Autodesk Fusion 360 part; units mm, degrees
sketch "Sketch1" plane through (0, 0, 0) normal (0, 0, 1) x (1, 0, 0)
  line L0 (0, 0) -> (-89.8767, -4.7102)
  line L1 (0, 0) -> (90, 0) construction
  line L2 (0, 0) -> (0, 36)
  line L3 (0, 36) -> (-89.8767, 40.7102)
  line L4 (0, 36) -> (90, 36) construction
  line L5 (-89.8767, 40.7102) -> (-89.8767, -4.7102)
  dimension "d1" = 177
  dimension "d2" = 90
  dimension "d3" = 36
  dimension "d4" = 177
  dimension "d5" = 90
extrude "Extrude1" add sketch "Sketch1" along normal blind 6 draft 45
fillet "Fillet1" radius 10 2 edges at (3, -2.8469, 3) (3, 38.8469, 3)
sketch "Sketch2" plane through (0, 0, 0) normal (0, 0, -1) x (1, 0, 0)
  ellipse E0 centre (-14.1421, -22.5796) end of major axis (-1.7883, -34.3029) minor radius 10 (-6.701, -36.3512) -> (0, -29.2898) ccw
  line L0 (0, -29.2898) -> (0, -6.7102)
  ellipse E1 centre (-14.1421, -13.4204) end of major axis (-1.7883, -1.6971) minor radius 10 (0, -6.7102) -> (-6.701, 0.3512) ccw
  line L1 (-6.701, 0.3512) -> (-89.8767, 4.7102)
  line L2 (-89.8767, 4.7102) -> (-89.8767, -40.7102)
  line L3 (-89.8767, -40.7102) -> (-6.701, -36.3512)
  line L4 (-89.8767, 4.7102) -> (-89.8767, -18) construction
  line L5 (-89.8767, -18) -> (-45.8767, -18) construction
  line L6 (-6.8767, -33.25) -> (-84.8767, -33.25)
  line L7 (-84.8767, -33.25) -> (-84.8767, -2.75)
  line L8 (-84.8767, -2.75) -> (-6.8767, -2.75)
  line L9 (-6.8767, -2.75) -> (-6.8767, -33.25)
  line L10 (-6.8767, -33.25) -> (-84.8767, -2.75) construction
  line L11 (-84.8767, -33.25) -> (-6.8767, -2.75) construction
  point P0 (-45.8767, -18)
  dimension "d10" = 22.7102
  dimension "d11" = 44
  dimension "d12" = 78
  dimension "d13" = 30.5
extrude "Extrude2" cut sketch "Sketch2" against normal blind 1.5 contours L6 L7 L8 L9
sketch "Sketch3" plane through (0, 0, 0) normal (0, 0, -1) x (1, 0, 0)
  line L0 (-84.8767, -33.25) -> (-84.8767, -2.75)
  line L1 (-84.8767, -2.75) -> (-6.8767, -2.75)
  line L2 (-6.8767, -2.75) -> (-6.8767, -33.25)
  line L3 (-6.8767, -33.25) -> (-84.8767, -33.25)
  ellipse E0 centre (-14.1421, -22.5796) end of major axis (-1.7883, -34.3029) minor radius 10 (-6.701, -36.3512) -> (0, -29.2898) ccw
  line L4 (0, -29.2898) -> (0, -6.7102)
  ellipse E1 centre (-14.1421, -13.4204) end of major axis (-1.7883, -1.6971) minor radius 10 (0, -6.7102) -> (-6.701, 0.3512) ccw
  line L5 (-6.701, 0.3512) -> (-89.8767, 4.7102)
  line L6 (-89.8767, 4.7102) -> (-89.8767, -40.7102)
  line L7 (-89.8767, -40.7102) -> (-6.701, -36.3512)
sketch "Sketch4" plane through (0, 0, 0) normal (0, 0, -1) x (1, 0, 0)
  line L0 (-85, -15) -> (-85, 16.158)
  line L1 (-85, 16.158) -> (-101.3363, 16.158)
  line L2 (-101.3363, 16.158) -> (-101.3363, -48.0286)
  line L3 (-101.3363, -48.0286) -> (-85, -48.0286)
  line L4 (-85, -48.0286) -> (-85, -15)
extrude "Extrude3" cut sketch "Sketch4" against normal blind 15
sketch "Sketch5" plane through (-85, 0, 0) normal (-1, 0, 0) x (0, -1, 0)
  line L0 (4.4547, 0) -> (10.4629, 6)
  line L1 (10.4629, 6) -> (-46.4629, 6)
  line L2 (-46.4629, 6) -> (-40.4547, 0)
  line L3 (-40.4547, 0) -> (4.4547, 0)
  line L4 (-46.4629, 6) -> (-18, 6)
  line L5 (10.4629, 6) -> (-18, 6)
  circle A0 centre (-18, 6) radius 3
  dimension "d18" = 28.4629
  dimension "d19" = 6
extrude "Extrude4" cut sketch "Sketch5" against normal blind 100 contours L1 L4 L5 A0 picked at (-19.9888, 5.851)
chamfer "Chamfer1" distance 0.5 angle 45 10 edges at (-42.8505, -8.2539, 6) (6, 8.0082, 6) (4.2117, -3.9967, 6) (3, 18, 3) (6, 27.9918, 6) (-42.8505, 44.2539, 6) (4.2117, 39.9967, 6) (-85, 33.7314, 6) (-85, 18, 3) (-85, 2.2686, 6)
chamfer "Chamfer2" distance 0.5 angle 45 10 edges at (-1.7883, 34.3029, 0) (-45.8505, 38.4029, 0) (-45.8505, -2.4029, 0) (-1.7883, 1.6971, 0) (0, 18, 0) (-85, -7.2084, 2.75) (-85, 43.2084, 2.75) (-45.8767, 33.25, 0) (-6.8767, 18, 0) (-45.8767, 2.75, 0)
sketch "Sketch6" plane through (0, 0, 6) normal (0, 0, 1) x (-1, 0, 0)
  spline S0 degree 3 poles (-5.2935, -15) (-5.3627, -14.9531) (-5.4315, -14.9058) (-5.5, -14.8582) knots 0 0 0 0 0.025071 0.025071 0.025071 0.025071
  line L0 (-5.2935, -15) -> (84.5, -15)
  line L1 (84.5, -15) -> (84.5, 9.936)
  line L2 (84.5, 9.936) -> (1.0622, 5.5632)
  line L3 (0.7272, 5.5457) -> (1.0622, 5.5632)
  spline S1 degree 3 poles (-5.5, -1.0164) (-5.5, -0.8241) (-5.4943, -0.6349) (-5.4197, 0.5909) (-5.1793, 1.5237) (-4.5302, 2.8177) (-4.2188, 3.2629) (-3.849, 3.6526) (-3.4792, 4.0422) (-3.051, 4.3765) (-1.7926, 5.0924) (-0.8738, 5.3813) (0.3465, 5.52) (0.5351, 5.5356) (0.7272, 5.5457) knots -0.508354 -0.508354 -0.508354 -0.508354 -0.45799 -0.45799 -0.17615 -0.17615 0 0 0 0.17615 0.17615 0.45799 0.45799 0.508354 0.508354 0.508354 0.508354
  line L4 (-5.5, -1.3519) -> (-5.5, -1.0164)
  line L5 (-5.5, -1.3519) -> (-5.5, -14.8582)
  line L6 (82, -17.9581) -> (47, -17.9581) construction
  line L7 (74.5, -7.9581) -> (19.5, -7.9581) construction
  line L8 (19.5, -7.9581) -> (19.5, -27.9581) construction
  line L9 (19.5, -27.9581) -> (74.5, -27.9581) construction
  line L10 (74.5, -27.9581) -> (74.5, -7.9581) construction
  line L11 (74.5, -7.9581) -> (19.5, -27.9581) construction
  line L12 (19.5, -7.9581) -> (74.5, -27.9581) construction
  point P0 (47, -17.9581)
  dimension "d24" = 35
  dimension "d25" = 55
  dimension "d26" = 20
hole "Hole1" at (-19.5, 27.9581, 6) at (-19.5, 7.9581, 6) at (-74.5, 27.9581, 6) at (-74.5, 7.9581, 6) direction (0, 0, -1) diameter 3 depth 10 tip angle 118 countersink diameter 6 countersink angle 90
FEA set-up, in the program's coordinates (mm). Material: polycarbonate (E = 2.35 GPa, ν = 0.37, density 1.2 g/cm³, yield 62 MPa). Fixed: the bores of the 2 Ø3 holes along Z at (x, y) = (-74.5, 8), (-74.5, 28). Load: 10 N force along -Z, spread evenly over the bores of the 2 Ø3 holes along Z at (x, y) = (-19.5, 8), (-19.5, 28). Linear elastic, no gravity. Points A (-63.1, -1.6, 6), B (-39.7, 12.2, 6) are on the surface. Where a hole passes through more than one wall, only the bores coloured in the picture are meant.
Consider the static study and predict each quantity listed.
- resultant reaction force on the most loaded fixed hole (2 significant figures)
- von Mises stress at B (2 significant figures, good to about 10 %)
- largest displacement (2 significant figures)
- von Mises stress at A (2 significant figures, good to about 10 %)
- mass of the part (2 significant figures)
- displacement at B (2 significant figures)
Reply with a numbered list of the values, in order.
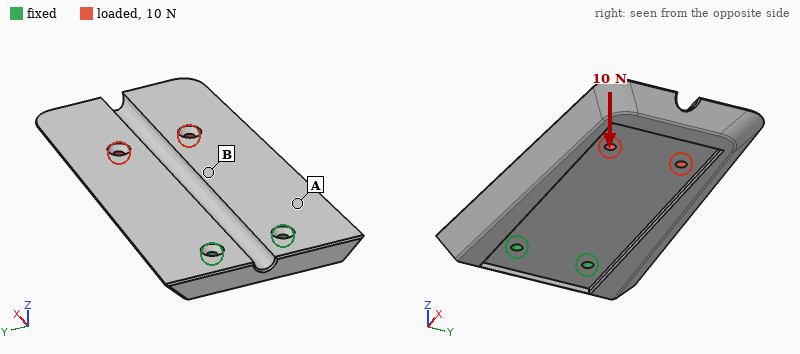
1. 8.5 N
2. 1.0 MPa
3. 1.1 mm
4. 2.0 MPa
5. 23 g
6. 0.36 mm
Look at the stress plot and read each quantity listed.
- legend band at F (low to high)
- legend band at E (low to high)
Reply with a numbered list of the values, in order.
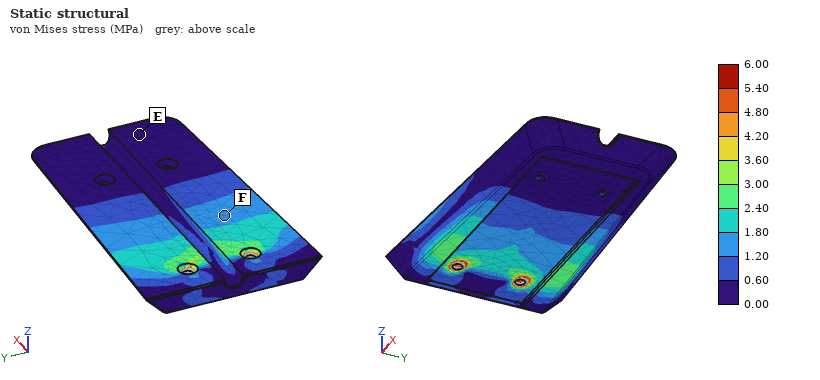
1. 1.20 to 1.80 MPa
2. 0.00 to 0.60 MPa
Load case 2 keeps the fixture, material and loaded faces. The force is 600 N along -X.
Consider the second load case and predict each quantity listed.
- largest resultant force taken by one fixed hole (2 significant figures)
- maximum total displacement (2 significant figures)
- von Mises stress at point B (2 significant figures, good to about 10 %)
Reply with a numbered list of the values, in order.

1. 300 N
2. 0.85 mm
3. 1.7 MPa
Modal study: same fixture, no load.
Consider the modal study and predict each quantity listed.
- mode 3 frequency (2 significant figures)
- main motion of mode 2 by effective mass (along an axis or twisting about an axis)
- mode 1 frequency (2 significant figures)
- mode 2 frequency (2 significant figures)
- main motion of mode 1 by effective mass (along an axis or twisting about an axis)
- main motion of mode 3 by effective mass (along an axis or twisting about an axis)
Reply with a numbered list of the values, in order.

1. 940 Hz
2. twisting about X
3. 170 Hz
4. 550 Hz
5. along Z
6. along Y
